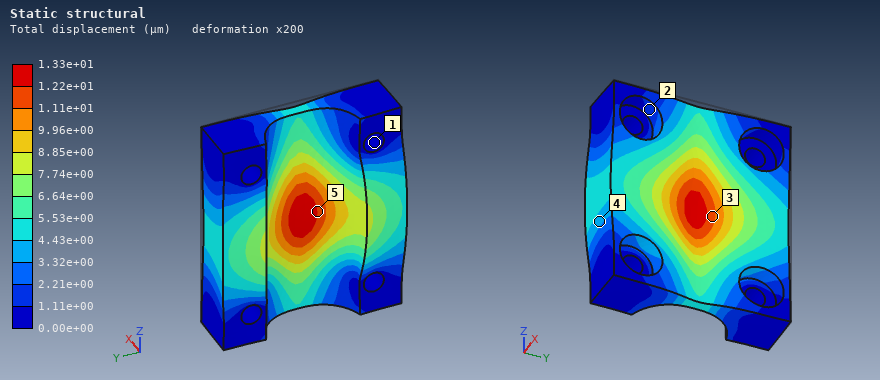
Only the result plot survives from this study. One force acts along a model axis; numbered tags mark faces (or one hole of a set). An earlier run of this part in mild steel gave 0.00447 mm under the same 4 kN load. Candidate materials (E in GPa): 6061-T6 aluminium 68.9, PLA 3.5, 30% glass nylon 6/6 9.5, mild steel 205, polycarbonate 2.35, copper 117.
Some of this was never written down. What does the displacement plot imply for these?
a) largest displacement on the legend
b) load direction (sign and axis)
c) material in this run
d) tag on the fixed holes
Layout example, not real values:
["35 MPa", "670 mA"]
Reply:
["1.33e+01 µm", "-X", "6061-T6 aluminium", "1"]
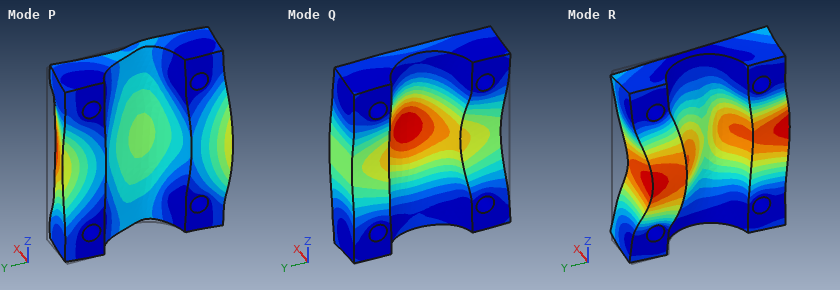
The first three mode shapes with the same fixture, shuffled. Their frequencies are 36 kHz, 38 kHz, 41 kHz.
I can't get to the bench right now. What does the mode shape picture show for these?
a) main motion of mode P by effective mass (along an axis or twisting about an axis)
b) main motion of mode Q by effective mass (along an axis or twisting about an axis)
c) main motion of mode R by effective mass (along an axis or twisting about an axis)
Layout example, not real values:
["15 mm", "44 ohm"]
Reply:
["along Y", "along X", "along Y"]
